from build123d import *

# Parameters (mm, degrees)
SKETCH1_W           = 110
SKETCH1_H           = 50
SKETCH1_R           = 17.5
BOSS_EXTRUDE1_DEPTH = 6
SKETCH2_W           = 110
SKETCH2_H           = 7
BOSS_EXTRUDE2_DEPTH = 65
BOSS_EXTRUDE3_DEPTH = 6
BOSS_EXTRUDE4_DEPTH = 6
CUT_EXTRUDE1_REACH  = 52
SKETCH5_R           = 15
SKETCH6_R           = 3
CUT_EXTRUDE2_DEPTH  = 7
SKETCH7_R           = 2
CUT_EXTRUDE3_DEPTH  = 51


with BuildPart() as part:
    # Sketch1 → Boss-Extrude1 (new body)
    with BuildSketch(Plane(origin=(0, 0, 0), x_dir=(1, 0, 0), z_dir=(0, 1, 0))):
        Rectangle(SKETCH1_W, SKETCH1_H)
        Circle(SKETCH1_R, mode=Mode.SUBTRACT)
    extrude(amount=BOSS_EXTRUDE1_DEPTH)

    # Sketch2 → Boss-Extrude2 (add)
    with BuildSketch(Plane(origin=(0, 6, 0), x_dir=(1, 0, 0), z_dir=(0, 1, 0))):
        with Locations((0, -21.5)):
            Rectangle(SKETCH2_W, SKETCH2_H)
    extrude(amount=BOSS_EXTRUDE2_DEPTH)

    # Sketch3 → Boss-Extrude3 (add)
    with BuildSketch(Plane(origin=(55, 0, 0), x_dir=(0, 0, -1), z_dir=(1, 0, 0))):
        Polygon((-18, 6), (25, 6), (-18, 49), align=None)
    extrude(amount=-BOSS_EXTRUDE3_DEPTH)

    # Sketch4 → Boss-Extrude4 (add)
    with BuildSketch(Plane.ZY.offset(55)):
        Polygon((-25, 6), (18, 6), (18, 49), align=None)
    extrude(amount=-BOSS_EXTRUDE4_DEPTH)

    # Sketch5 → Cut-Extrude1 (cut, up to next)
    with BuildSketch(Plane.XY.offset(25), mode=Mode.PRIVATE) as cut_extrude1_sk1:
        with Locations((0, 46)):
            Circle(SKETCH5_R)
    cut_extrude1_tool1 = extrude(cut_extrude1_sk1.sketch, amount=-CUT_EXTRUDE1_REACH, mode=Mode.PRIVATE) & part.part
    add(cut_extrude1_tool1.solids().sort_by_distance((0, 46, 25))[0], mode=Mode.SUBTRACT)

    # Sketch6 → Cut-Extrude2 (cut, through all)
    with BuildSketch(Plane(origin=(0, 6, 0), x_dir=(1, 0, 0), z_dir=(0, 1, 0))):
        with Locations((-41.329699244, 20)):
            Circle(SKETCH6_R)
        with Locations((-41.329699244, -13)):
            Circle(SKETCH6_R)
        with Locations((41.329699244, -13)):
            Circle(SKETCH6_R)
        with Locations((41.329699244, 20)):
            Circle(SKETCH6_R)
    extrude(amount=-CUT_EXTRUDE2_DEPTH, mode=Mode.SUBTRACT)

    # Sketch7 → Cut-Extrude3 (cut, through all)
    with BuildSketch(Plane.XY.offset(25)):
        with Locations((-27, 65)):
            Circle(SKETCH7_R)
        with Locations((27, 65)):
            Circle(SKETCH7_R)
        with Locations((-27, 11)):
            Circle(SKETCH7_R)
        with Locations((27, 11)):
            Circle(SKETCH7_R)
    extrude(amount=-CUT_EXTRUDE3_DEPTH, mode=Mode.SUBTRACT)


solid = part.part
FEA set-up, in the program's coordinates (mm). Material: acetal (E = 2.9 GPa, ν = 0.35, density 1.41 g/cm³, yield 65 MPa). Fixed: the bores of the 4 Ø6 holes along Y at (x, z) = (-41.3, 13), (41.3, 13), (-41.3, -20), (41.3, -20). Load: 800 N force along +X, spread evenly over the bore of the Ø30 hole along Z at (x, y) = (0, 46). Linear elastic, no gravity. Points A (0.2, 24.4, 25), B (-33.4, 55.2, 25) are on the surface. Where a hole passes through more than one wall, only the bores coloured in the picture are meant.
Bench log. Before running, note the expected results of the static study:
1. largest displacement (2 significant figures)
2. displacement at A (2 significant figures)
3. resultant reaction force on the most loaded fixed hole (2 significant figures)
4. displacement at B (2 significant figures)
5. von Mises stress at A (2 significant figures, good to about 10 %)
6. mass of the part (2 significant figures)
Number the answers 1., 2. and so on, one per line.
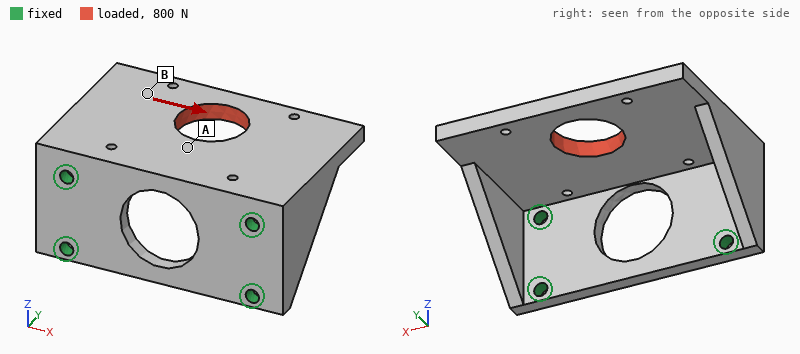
1. 0.25 mm
2. 0.066 mm
3. 590 N
4. 0.17 mm
5. 3.4 MPa
6. 120 g
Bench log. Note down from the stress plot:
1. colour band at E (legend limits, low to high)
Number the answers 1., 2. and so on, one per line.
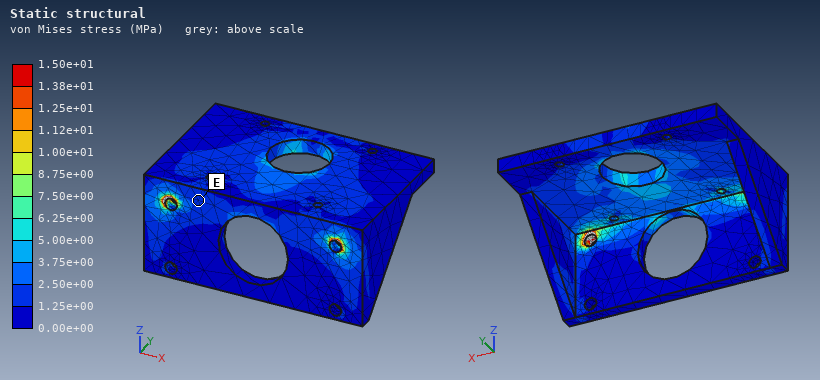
1. 1.25e+00 to 2.50e+00 MPa
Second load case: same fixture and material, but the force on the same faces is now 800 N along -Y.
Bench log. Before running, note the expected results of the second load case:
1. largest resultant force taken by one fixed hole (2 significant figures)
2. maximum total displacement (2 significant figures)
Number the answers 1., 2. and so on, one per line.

1. 470 N
2. 0.23 mm
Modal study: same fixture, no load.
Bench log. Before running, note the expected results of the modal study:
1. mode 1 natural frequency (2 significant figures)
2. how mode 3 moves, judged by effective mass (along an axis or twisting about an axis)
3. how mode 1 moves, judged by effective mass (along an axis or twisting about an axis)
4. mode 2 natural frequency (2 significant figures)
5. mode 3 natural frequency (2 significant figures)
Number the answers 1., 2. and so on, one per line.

1. 530 Hz
2. along X
3. along Z
4. 980 Hz
5. 1600 Hz
